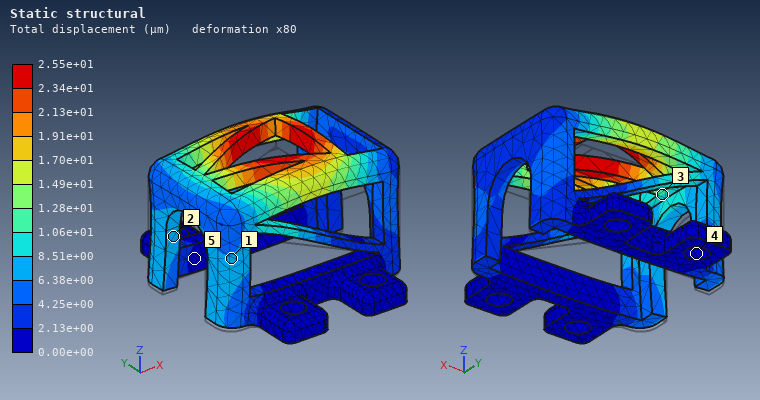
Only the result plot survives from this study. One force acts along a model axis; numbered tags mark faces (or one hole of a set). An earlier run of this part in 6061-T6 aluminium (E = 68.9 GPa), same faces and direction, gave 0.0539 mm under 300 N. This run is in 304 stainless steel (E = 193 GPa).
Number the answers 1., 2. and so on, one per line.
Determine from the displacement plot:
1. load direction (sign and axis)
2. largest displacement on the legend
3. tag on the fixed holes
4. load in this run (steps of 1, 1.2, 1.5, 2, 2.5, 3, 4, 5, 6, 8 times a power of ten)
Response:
1. +Z
2. 2.55e+01 µm
3. 4
4. 400 N
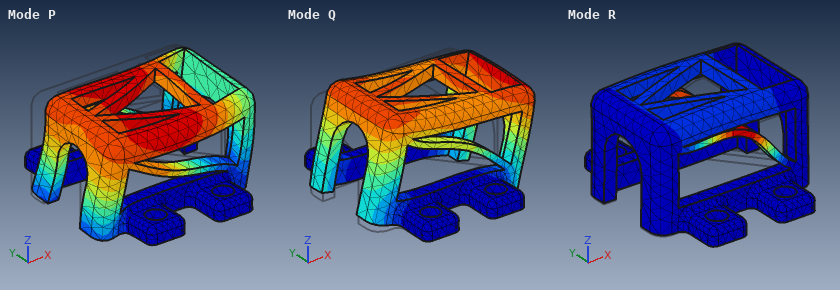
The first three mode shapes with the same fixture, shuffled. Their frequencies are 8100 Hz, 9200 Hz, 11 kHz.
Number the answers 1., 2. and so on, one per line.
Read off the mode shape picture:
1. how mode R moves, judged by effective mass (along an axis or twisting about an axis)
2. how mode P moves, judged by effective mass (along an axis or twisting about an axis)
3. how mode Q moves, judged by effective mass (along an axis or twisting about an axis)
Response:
1. along Z
2. along Y
3. along X
